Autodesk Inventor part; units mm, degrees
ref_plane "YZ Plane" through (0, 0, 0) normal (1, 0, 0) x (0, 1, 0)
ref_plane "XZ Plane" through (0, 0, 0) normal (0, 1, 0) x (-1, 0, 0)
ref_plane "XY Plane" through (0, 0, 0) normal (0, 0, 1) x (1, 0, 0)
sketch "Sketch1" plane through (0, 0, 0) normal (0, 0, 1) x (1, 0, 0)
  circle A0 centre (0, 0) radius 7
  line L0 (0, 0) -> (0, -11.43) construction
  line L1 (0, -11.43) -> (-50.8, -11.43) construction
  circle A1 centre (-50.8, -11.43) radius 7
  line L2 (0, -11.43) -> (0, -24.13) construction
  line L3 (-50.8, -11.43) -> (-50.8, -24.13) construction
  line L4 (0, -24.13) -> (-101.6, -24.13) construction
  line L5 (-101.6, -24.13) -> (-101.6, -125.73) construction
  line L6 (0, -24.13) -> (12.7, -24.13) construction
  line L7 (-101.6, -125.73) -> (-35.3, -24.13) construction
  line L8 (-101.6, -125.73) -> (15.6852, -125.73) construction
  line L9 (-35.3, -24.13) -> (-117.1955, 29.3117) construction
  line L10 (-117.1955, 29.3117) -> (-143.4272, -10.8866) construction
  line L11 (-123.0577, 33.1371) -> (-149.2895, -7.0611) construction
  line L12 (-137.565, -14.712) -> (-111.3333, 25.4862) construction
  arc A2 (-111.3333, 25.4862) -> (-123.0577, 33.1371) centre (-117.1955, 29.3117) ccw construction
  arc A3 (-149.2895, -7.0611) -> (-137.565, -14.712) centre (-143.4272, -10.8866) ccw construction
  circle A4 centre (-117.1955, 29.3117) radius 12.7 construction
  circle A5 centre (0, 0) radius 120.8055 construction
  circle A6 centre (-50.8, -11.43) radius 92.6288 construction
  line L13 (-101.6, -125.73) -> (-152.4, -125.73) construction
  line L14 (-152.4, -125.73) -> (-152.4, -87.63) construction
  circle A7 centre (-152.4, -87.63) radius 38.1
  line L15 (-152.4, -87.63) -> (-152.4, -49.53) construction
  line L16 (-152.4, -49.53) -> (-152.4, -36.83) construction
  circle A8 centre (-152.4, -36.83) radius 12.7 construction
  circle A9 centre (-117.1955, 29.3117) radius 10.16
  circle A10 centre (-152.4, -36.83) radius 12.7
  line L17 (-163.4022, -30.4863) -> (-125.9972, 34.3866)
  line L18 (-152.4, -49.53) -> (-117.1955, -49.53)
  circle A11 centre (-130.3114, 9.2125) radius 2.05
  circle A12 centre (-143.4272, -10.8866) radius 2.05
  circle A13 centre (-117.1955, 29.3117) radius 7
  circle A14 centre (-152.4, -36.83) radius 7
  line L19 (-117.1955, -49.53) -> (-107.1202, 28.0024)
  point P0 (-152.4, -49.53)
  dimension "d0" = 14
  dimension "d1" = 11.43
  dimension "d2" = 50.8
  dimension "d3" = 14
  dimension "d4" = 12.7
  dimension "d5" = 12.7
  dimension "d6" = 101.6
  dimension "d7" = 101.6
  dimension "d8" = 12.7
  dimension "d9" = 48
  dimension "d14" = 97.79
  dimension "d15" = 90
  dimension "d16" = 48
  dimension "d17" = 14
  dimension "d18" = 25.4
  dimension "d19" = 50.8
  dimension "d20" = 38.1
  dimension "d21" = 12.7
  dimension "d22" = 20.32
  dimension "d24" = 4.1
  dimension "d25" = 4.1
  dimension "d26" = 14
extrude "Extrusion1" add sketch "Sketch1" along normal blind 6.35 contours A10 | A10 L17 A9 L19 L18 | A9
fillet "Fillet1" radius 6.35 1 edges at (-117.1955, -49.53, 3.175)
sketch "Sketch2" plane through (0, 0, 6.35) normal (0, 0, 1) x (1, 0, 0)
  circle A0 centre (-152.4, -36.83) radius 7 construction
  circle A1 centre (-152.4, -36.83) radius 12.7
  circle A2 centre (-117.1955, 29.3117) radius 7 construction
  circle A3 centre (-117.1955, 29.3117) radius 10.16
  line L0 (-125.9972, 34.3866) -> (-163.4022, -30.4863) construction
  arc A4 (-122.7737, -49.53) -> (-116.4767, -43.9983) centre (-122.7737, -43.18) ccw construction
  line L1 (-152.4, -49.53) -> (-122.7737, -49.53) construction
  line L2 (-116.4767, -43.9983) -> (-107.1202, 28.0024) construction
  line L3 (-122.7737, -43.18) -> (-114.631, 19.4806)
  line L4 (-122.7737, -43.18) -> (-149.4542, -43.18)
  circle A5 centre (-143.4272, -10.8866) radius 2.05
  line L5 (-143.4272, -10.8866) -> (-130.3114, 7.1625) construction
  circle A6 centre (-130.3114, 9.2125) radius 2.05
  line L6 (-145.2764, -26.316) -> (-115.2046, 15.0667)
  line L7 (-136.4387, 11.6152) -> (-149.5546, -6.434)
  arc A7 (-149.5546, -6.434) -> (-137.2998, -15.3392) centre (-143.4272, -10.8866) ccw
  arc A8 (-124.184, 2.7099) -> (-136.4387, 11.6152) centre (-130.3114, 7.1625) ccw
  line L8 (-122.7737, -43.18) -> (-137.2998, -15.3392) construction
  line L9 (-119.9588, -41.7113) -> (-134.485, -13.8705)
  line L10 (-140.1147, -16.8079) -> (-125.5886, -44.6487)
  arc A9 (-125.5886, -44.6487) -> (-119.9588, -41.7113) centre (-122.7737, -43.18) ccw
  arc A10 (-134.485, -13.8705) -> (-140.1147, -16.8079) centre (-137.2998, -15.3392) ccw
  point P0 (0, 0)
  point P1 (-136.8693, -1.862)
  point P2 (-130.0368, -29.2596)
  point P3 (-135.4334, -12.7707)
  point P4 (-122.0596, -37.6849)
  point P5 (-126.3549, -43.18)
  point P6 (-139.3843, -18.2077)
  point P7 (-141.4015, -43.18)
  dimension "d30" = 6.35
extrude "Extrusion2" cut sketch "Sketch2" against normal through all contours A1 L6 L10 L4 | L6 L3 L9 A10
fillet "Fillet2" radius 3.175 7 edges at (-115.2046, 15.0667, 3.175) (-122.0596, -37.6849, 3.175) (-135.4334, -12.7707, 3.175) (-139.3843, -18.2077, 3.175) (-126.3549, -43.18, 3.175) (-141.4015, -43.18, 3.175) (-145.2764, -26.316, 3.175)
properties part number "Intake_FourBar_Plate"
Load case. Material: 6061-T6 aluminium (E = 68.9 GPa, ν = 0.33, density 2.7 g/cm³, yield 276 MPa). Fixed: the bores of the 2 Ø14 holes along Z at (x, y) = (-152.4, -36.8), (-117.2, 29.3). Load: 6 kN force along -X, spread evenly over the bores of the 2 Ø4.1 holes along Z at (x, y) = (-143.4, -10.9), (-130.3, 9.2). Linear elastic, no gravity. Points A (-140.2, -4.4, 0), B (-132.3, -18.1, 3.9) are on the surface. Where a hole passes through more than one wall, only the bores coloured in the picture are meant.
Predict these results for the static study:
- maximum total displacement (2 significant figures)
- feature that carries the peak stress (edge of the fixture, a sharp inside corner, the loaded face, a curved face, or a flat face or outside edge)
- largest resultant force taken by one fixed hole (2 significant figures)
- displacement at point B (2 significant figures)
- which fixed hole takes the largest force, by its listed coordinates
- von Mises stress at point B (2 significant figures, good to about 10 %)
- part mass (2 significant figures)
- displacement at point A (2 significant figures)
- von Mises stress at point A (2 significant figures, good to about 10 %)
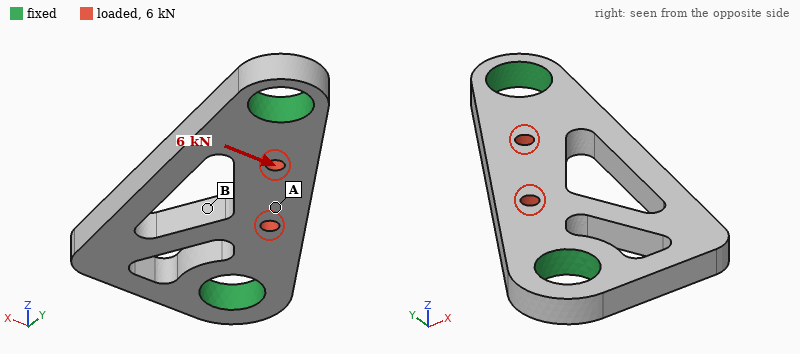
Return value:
37 µm
edge of the fixture
3.5 kN
27 µm
(-117.2, 29.3)
45 MPa
39 g
37 µm
17 MPa
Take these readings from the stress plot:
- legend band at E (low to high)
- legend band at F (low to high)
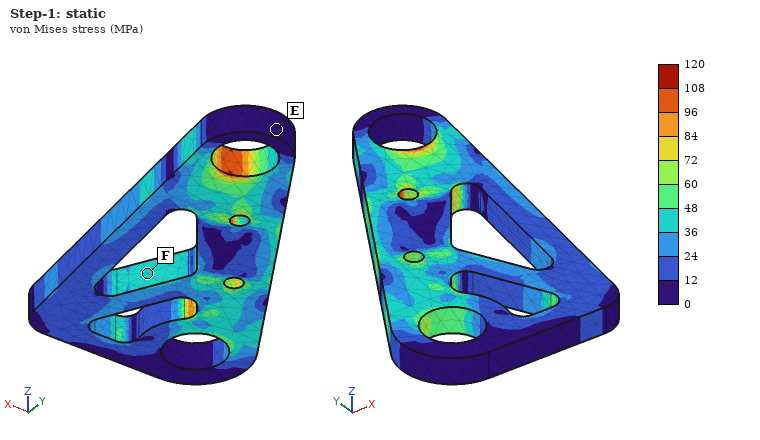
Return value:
0 to 12 MPa
36 to 48 MPa
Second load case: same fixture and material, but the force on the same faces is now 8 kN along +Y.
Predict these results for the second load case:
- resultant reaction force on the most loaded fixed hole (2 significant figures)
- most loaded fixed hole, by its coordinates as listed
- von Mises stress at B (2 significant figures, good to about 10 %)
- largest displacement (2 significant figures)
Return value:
4.5 kN
(-117.2, 29.3)
43 MPa
29 µm
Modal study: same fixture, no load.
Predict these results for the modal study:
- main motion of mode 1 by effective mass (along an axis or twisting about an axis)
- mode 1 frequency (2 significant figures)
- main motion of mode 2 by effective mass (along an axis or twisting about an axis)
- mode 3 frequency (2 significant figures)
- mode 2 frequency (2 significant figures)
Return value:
along Z
4100 Hz
along Z
9700 Hz
7700 Hz
